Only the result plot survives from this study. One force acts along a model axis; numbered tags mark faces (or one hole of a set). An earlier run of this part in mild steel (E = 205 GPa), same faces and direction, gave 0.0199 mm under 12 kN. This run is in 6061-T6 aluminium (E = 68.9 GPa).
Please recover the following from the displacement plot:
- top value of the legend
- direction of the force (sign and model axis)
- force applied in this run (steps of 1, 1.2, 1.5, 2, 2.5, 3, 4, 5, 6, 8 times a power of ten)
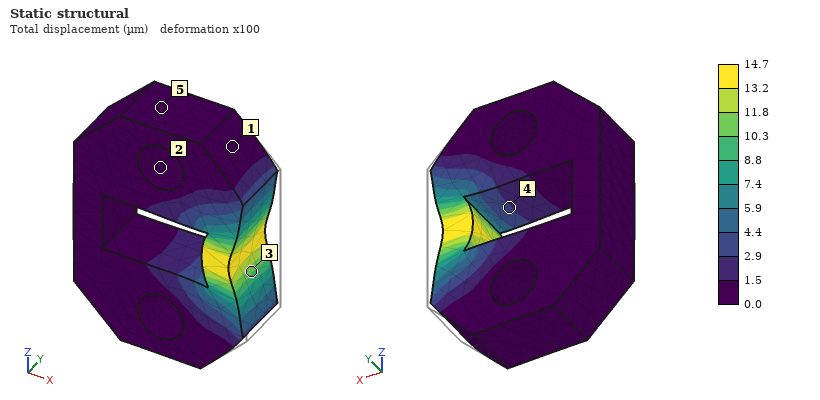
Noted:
14.7 µm
-X
3 kN
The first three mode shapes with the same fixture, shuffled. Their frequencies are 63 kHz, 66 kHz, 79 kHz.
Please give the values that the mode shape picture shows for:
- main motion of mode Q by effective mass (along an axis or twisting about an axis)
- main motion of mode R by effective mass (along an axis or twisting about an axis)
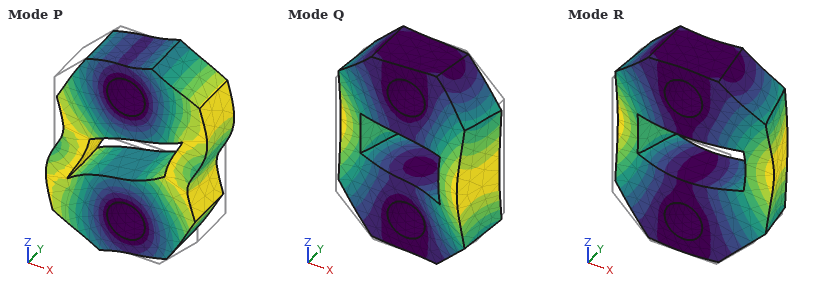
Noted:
twisting about Z
along Y
